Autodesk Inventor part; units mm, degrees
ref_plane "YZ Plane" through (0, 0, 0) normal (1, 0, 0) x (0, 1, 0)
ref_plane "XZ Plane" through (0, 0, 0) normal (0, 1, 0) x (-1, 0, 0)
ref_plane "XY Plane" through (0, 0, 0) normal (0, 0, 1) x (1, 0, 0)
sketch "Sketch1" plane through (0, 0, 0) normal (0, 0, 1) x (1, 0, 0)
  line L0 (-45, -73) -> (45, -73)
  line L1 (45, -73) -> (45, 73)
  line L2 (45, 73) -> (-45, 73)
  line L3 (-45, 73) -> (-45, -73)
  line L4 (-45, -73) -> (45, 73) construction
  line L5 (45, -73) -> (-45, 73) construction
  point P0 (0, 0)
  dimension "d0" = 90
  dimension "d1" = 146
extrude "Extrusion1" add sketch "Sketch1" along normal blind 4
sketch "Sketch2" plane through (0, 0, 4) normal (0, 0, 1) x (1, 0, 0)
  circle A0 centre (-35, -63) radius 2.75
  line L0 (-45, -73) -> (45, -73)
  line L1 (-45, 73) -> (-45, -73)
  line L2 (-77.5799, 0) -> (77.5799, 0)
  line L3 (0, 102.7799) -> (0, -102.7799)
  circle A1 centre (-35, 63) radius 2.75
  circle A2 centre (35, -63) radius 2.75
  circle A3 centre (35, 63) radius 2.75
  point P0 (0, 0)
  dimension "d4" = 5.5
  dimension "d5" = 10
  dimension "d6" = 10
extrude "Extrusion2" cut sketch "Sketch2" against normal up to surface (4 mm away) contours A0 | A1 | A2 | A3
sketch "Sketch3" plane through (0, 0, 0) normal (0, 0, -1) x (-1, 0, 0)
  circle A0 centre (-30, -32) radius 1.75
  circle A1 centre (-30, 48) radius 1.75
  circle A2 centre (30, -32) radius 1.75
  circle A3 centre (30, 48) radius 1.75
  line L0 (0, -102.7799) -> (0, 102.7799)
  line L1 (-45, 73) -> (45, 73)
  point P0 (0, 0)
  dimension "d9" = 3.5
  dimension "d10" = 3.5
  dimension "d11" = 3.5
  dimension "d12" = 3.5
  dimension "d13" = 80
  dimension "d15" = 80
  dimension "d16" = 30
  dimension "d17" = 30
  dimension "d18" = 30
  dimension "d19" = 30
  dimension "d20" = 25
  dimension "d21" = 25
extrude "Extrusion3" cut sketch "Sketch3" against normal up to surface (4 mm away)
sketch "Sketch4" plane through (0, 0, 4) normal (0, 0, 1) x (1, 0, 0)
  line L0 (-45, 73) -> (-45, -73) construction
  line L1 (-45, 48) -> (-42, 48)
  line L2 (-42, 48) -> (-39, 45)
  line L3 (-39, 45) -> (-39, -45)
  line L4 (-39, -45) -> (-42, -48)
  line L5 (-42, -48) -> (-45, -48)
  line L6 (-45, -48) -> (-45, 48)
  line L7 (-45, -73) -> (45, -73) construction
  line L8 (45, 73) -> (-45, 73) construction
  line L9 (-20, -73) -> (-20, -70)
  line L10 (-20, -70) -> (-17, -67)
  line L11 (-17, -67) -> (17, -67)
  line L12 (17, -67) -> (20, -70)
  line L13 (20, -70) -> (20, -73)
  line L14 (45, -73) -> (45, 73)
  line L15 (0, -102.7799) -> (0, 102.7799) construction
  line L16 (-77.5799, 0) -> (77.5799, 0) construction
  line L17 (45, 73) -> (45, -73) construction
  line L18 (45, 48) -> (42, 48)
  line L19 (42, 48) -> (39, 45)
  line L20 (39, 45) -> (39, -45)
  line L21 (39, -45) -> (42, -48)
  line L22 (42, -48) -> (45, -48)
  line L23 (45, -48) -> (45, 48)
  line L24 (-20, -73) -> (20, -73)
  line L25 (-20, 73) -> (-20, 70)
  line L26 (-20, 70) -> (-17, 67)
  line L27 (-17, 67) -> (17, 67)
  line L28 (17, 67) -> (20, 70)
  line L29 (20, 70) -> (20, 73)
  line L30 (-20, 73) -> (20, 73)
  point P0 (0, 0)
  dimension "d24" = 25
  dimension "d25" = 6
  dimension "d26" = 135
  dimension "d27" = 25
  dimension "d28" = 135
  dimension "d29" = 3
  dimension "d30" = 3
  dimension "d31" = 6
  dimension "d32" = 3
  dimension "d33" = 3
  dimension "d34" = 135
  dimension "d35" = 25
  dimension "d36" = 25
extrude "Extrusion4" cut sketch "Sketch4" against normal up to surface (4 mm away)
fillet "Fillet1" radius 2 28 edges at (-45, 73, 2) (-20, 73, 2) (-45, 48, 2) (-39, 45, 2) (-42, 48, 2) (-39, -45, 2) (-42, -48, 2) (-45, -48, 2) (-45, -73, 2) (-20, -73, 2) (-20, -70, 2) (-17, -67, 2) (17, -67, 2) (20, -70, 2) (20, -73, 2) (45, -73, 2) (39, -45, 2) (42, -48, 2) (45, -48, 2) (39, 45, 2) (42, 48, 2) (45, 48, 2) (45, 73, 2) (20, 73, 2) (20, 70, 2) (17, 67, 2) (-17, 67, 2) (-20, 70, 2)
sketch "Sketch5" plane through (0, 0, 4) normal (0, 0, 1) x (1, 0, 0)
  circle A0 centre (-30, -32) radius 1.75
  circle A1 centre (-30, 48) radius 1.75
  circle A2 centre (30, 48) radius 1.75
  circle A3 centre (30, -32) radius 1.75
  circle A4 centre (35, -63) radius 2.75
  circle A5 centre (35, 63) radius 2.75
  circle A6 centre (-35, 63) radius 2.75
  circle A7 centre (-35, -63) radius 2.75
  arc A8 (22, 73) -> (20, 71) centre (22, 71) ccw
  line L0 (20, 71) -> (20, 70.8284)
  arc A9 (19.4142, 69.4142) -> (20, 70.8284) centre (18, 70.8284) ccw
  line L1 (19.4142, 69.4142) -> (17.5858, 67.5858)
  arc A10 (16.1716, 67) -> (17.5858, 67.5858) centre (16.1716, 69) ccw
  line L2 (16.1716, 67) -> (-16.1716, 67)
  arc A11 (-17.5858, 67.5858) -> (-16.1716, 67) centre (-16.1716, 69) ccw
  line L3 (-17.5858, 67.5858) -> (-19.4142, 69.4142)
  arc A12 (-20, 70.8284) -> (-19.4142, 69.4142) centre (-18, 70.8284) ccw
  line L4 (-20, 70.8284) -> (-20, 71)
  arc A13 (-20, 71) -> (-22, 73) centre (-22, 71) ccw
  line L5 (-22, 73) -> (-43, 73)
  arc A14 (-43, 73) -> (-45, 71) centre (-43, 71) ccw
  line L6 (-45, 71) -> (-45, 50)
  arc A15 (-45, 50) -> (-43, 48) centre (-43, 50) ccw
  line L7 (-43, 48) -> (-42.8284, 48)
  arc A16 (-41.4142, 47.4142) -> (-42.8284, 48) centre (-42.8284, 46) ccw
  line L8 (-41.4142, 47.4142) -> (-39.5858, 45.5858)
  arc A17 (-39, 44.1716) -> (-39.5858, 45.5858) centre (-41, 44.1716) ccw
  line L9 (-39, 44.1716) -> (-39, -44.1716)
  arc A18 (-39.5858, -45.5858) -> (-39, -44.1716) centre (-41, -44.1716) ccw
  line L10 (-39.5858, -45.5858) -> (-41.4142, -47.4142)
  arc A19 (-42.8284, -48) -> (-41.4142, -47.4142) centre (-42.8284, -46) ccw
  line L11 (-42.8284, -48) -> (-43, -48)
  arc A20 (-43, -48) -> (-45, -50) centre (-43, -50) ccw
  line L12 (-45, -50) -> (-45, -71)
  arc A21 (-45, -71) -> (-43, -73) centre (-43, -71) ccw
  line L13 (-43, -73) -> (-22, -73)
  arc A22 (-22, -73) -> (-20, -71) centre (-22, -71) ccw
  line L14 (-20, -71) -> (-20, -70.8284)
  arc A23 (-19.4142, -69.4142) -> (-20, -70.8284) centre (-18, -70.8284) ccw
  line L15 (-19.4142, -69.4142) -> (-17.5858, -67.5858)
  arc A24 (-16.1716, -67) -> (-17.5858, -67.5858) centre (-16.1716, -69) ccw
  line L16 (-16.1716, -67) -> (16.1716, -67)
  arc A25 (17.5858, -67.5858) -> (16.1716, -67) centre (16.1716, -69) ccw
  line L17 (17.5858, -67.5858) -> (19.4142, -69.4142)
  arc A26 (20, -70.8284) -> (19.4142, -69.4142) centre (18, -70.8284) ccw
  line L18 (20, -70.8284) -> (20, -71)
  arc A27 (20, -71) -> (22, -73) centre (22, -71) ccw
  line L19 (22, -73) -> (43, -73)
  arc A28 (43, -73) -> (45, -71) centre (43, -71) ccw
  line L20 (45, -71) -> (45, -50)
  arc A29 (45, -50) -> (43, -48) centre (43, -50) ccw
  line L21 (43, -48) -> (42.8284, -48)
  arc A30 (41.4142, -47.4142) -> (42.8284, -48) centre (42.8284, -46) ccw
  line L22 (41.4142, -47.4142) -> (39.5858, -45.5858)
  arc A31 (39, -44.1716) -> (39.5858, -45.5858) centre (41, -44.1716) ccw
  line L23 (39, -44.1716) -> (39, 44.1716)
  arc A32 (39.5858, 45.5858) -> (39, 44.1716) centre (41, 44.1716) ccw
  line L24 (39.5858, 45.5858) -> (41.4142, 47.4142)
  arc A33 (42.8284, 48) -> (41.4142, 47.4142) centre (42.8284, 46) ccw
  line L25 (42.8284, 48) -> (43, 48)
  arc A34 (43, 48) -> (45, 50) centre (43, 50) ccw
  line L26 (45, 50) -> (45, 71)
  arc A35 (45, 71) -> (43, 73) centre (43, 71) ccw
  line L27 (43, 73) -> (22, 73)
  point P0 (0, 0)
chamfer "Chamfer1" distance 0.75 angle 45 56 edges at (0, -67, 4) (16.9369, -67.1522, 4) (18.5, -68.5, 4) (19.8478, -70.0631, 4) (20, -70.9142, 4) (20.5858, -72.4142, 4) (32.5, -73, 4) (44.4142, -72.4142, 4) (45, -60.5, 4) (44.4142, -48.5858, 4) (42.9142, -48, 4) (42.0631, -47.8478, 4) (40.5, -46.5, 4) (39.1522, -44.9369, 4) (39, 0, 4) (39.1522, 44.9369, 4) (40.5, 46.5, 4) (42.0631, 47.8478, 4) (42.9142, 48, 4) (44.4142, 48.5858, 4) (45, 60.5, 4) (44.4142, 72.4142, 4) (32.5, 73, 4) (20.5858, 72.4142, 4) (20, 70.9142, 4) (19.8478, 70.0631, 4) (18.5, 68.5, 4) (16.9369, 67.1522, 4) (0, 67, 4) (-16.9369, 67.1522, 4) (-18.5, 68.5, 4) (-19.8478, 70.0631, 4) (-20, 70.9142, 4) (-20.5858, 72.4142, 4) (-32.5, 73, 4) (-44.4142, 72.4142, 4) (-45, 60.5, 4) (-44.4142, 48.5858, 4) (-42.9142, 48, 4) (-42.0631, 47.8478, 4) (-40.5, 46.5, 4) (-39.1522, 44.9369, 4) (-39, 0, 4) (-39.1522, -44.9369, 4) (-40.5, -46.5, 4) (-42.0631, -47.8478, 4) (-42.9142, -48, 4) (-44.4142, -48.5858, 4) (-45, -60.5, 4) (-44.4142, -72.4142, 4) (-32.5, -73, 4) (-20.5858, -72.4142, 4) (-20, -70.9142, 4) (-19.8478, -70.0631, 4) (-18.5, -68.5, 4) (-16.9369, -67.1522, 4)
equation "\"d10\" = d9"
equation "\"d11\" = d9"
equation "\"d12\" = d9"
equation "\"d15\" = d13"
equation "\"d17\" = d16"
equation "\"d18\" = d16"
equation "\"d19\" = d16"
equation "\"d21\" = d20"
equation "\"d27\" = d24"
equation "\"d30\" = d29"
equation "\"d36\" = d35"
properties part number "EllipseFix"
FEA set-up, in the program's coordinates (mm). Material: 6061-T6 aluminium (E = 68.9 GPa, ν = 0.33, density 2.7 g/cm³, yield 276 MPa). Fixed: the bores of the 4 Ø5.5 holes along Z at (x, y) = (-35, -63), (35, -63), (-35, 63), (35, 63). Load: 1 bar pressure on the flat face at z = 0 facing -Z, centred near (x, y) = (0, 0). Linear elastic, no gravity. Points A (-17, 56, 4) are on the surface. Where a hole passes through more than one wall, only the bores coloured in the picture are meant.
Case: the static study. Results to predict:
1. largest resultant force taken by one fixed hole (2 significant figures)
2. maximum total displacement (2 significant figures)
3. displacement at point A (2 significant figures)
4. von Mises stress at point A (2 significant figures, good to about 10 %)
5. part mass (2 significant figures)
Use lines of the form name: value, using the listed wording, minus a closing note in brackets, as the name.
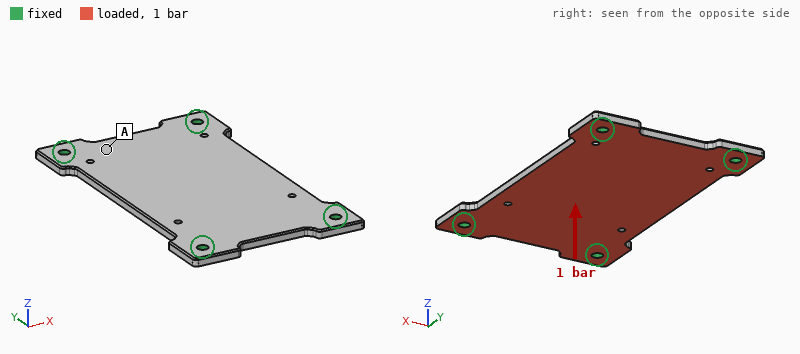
largest resultant force taken by one fixed hole: 290 N
maximum total displacement: 0.22 mm
displacement at point A: 0.036 mm
von Mises stress at point A: 17 MPa
part mass: 120 g
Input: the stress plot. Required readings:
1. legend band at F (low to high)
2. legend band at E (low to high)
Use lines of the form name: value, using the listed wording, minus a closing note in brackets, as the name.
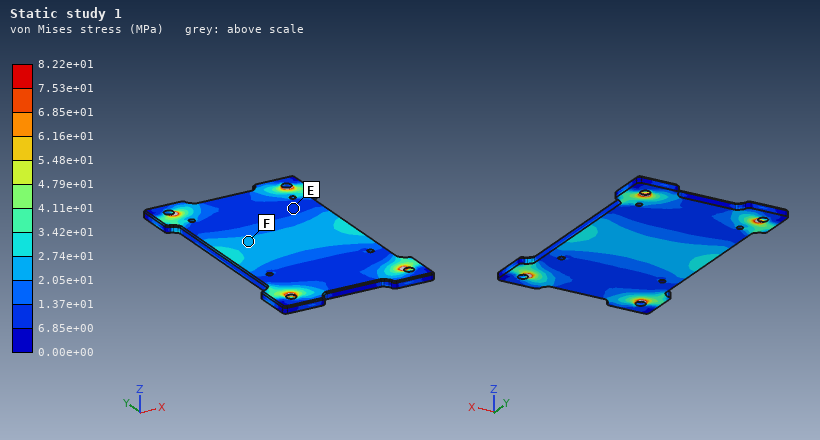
legend band at F: 2.05e+01 to 2.74e+01 MPa
legend band at E: 6.85e+00 to 1.37e+01 MPa
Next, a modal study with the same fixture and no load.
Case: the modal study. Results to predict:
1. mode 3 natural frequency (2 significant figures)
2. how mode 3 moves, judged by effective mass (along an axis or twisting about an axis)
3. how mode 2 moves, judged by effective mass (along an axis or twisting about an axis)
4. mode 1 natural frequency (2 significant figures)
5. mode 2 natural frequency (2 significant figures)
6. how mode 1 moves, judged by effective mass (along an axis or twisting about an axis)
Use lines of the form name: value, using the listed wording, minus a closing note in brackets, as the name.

mode 3 natural frequency: 3100 Hz
how mode 3 moves, judged by effective mass: twisting about X
how mode 2 moves, judged by effective mass: twisting about Y
mode 1 natural frequency: 1200 Hz
mode 2 natural frequency: 2000 Hz
how mode 1 moves, judged by effective mass: along Z
